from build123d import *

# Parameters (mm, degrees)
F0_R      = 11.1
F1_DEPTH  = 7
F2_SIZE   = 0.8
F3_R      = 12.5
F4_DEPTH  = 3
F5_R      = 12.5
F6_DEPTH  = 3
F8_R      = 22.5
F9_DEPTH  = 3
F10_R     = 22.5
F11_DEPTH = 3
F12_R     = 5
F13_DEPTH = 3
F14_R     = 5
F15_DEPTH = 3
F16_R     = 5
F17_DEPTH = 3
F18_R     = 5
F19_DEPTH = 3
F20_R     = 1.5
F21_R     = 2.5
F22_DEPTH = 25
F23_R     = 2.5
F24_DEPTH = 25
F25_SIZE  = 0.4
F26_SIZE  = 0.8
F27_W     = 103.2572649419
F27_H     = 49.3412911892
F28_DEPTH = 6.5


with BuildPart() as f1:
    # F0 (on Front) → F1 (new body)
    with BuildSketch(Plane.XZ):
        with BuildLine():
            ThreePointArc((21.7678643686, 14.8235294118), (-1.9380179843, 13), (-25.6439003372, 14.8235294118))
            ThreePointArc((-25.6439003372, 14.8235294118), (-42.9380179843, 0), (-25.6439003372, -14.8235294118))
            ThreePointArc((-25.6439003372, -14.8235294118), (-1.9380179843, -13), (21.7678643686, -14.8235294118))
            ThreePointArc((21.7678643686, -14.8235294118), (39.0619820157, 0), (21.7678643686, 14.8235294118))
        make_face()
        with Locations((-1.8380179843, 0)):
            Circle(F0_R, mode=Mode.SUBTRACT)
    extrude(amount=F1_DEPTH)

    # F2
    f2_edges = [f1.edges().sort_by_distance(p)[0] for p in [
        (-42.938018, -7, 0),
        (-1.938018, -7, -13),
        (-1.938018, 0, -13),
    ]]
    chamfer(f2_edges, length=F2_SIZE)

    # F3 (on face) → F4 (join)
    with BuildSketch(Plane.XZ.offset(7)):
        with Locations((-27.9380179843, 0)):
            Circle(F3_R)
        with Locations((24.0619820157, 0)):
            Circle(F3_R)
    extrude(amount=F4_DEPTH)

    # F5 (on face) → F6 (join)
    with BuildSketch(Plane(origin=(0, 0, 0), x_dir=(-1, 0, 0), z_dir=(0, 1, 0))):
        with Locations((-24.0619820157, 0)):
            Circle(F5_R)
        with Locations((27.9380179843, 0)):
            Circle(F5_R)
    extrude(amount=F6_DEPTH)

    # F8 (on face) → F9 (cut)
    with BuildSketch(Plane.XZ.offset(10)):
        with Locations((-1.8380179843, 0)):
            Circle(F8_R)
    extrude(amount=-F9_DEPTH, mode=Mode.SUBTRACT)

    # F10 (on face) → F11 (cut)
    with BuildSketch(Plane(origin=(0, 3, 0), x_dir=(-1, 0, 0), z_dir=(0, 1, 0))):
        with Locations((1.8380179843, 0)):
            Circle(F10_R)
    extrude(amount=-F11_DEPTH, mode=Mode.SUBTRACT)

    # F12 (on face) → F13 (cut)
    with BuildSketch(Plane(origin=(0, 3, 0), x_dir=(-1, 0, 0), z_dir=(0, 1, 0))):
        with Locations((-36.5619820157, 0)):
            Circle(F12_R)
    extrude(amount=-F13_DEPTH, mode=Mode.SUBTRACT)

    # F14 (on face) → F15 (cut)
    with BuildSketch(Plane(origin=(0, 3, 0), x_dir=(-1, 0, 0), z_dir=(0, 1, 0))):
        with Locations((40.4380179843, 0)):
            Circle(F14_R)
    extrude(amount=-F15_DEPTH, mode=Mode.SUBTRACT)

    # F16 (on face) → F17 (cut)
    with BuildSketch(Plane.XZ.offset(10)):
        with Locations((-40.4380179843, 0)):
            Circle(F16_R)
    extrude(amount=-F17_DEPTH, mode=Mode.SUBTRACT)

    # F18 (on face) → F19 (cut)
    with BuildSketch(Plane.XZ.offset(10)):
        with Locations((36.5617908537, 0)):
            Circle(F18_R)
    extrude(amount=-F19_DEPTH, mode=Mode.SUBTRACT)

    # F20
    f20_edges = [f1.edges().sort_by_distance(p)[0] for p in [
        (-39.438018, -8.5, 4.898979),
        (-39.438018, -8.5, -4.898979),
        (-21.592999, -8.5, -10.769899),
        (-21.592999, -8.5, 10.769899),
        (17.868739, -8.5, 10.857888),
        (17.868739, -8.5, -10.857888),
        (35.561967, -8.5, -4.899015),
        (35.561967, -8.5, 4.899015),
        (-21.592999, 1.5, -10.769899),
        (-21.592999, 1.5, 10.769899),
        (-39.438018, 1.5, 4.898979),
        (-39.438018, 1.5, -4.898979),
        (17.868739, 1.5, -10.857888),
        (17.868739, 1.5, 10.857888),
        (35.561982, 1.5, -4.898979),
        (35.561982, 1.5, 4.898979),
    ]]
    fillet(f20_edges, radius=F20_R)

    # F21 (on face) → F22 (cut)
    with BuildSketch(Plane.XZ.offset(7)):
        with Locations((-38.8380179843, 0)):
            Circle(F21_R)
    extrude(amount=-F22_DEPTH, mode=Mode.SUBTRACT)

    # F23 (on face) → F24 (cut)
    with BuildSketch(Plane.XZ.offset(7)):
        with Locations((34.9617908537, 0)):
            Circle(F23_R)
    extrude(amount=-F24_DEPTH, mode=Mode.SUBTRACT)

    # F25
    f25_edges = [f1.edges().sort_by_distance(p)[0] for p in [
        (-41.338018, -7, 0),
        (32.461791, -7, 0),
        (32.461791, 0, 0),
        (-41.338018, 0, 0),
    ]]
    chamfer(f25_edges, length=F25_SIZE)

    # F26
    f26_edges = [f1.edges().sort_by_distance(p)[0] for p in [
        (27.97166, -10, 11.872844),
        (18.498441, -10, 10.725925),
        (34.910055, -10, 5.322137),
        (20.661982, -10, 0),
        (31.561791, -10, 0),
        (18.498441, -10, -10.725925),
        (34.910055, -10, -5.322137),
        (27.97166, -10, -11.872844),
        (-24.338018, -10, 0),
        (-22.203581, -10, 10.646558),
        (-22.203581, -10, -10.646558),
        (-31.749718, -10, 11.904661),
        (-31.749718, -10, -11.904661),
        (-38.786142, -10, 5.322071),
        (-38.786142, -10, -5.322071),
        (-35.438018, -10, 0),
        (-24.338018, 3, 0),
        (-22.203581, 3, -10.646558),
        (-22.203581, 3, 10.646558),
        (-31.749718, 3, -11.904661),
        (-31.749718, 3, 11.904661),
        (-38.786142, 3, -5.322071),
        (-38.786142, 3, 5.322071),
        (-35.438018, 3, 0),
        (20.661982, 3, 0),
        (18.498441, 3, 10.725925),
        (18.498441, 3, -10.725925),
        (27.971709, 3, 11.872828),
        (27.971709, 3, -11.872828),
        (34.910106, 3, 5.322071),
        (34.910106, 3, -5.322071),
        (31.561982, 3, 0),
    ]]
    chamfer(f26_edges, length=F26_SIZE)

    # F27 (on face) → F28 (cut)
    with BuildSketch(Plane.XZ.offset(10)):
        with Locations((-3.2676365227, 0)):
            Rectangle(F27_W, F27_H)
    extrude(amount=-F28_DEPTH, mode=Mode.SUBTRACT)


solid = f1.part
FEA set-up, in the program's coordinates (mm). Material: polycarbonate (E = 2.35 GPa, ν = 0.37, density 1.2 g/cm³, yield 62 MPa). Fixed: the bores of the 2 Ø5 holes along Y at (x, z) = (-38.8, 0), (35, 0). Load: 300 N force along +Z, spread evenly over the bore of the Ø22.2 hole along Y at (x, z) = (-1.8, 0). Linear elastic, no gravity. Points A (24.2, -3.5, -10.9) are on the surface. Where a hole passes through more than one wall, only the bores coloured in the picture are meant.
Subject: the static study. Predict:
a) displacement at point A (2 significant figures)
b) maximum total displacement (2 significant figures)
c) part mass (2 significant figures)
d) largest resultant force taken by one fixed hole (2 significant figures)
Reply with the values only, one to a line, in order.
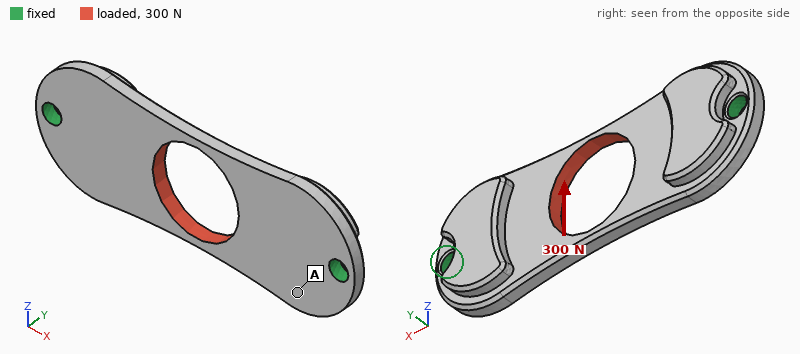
0.11 mm
0.28 mm
9.3 g
150 N
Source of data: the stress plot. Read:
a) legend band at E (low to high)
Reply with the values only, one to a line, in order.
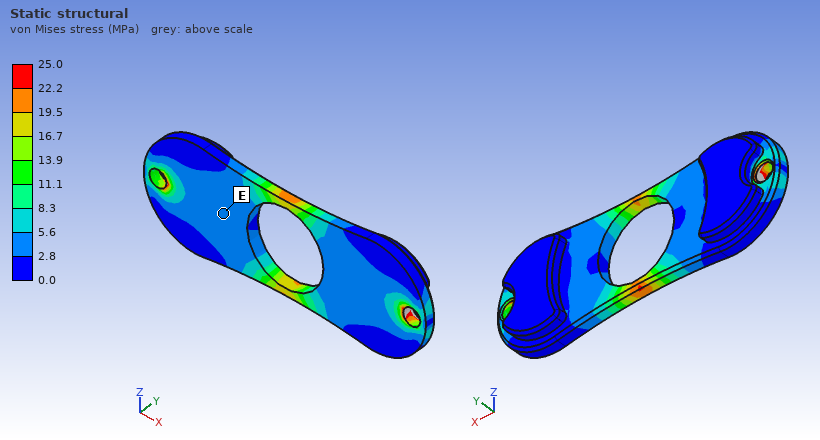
2.8 to 5.6 MPa
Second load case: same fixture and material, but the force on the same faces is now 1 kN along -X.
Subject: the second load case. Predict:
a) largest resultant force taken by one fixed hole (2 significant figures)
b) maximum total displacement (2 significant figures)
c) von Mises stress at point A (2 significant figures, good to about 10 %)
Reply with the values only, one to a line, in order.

500 N
0.12 mm
4.9 MPa
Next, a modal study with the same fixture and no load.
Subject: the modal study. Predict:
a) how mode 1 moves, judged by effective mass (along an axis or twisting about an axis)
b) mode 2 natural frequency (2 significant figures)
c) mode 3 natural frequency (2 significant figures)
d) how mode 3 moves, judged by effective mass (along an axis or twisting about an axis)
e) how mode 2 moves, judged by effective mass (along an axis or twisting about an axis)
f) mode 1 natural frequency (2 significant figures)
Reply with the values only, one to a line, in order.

along Y
1900 Hz
2100 Hz
twisting about Z
twisting about X
1200 Hz
